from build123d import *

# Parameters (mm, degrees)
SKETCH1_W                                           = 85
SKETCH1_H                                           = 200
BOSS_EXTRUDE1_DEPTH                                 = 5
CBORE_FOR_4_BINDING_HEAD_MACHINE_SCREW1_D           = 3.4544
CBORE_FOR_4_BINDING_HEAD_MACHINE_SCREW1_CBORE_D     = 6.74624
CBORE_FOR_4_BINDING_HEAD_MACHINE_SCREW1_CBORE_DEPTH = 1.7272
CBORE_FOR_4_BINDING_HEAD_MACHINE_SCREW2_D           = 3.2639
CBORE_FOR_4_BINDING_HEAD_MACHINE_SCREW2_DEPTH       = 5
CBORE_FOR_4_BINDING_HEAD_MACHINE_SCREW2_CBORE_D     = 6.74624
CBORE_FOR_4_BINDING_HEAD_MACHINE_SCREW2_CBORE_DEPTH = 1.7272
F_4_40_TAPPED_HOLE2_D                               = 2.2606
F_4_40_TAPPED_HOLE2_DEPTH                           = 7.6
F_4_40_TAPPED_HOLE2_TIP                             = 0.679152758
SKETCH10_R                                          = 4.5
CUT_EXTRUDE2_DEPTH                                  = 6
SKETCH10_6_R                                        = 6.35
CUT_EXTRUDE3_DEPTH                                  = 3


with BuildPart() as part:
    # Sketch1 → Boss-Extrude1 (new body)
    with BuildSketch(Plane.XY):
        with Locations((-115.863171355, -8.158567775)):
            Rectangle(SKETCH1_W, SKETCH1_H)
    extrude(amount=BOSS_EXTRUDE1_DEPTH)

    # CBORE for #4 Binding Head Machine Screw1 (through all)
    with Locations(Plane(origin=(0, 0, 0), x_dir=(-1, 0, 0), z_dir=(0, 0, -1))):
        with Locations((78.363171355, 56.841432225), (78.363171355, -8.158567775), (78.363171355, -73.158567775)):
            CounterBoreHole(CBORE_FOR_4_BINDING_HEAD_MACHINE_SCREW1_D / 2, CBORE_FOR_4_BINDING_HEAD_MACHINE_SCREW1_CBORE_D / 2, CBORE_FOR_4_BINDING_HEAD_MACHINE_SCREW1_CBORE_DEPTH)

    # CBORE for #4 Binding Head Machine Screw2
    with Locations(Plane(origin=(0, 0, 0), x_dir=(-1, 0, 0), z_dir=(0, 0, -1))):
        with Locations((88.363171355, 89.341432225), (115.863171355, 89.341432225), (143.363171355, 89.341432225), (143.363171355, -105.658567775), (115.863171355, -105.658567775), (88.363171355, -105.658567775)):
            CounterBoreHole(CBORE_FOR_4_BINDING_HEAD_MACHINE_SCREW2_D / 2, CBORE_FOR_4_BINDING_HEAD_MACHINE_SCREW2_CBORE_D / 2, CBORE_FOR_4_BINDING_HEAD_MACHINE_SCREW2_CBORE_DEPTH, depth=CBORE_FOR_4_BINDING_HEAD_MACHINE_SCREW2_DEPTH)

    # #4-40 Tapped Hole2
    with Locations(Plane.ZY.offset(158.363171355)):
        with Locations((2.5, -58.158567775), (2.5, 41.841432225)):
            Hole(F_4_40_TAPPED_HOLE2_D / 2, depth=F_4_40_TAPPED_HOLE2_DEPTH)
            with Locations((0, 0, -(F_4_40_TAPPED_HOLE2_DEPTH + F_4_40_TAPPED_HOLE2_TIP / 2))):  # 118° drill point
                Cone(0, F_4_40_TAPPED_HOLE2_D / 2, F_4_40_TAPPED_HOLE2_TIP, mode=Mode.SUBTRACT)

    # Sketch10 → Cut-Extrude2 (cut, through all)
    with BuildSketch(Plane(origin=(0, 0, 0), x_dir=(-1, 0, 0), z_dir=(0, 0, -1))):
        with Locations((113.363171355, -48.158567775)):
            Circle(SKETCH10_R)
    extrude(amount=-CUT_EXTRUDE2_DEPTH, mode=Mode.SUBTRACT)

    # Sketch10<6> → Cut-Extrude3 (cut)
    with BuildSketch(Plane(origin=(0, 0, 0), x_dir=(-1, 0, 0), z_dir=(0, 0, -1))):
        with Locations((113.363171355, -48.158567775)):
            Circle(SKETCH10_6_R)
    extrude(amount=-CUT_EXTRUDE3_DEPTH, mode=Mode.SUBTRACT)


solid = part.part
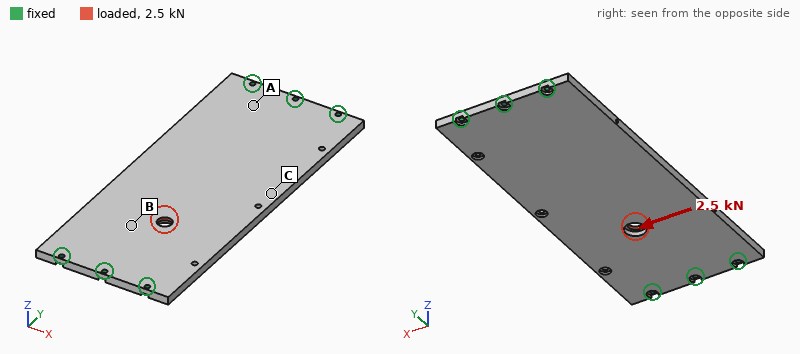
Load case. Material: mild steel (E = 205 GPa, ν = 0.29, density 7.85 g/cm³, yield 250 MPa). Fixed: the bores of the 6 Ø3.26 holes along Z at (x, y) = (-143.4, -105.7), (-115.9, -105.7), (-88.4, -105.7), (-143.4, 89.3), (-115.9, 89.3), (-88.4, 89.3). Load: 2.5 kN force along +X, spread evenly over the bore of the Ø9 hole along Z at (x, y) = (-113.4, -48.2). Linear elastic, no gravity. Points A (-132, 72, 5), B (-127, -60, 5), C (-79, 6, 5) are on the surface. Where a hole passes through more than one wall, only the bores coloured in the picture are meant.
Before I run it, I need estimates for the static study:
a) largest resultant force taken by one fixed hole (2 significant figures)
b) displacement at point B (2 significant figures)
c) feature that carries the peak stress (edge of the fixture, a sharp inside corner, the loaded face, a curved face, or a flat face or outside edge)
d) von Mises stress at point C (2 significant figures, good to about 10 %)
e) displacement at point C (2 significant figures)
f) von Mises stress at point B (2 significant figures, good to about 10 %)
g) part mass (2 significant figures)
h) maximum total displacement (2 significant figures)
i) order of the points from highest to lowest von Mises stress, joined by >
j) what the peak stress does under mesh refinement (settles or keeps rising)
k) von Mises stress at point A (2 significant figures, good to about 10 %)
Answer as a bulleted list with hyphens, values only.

- 890 N
- 7.4 µm
- edge of the fixture
- 4.7 MPa
- 13 µm
- 16 MPa
- 660 g
- 19 µm
- B > A > C
- keeps rising
- 7.7 MPa
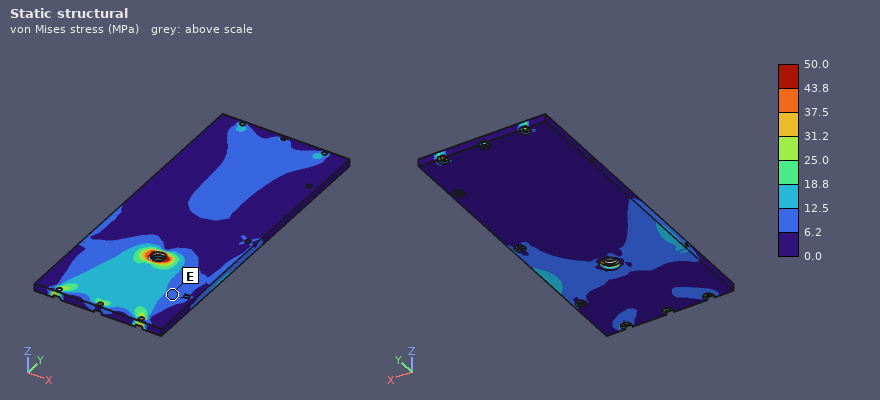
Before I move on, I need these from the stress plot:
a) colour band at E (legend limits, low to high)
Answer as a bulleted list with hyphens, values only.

- 6.2 to 12.5 MPa
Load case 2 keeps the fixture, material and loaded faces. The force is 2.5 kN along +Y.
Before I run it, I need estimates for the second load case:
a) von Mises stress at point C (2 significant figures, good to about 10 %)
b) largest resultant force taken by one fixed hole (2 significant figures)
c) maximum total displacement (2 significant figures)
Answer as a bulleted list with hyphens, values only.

- 4.2 MPa
- 580 N
- 13 µm
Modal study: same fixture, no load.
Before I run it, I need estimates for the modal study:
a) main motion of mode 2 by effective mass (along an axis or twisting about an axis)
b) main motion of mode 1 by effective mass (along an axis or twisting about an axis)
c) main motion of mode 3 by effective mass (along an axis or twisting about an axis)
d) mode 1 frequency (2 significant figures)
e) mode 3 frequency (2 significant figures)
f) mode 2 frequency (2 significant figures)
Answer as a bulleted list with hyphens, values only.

- twisting about Y
- along Z
- twisting about X
- 570 Hz
- 1600 Hz
- 1100 Hz
